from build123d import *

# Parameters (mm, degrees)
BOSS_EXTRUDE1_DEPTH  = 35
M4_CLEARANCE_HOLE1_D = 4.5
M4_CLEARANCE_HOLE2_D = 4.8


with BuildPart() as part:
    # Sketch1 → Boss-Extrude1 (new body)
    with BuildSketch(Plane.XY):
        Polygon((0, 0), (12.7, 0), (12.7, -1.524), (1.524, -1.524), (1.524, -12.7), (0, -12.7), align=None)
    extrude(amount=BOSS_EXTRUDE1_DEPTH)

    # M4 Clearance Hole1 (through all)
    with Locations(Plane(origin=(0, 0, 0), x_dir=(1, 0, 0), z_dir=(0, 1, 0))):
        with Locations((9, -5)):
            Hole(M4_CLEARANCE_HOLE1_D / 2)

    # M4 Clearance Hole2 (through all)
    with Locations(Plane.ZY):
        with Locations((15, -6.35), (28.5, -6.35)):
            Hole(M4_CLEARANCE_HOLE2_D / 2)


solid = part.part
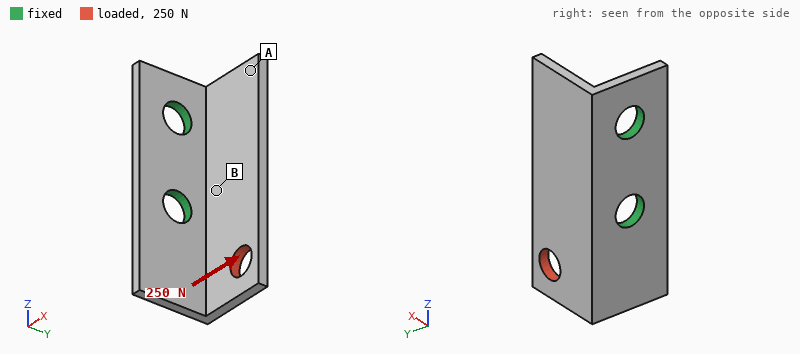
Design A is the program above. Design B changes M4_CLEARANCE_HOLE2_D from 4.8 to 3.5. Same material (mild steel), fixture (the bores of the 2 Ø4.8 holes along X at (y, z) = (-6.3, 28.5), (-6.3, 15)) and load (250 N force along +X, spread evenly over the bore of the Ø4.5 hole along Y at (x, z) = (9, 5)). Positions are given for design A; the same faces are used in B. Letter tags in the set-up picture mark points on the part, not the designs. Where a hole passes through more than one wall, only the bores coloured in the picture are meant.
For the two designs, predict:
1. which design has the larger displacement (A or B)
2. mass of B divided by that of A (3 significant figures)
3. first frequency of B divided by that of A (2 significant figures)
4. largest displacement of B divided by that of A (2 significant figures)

B
1.02
0.92
1.4
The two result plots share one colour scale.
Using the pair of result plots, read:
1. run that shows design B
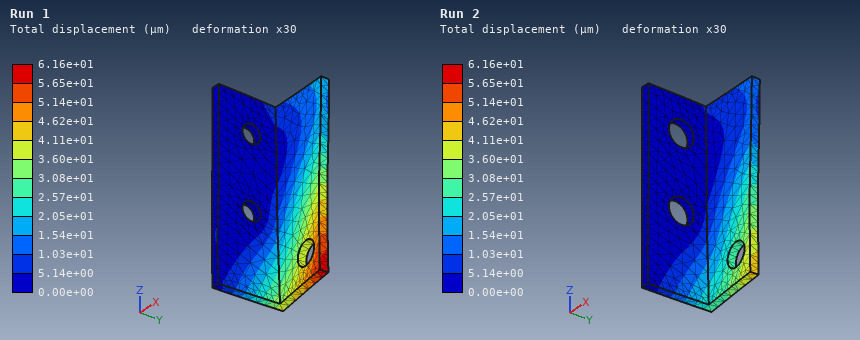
Run 1
